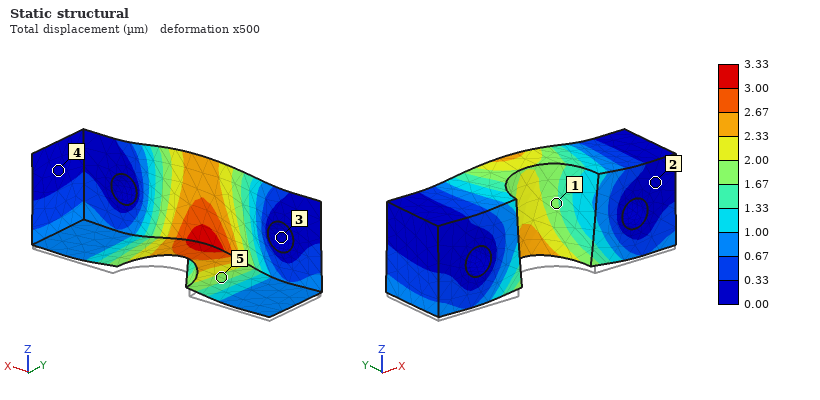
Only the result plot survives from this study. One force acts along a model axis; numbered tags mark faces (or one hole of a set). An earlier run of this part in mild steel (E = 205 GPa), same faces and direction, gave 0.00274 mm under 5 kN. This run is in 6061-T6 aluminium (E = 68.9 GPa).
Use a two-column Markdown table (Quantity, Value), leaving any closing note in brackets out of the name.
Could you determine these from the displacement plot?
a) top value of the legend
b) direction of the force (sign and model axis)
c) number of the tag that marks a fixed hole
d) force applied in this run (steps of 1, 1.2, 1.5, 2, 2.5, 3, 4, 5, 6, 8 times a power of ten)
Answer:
| Quantity | Value |
|---|---|
| top value of the legend | 3.33 µm |
| direction of the force | +Z |
| number of the tag that marks a fixed hole | 3 |
| force applied in this run | 2 kN |
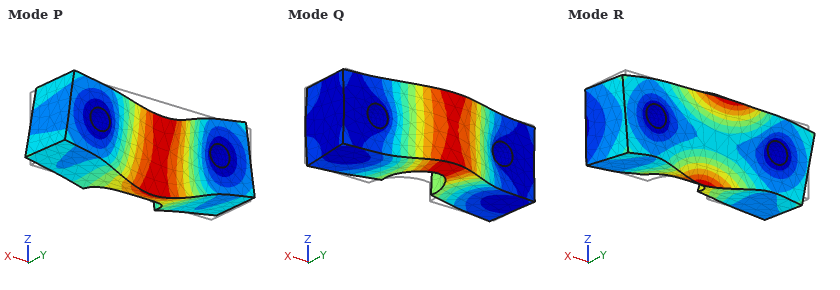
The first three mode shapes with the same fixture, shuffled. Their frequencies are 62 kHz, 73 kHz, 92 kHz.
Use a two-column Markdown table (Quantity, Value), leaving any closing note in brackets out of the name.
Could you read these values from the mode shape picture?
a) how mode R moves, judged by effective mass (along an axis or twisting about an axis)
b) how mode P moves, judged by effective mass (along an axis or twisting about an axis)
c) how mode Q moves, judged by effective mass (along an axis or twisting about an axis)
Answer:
| Quantity | Value |
|---|---|
| how mode R moves, judged by effective mass | twisting about X |
| how mode P moves, judged by effective mass | along Z |
| how mode Q moves, judged by effective mass | along Y |
